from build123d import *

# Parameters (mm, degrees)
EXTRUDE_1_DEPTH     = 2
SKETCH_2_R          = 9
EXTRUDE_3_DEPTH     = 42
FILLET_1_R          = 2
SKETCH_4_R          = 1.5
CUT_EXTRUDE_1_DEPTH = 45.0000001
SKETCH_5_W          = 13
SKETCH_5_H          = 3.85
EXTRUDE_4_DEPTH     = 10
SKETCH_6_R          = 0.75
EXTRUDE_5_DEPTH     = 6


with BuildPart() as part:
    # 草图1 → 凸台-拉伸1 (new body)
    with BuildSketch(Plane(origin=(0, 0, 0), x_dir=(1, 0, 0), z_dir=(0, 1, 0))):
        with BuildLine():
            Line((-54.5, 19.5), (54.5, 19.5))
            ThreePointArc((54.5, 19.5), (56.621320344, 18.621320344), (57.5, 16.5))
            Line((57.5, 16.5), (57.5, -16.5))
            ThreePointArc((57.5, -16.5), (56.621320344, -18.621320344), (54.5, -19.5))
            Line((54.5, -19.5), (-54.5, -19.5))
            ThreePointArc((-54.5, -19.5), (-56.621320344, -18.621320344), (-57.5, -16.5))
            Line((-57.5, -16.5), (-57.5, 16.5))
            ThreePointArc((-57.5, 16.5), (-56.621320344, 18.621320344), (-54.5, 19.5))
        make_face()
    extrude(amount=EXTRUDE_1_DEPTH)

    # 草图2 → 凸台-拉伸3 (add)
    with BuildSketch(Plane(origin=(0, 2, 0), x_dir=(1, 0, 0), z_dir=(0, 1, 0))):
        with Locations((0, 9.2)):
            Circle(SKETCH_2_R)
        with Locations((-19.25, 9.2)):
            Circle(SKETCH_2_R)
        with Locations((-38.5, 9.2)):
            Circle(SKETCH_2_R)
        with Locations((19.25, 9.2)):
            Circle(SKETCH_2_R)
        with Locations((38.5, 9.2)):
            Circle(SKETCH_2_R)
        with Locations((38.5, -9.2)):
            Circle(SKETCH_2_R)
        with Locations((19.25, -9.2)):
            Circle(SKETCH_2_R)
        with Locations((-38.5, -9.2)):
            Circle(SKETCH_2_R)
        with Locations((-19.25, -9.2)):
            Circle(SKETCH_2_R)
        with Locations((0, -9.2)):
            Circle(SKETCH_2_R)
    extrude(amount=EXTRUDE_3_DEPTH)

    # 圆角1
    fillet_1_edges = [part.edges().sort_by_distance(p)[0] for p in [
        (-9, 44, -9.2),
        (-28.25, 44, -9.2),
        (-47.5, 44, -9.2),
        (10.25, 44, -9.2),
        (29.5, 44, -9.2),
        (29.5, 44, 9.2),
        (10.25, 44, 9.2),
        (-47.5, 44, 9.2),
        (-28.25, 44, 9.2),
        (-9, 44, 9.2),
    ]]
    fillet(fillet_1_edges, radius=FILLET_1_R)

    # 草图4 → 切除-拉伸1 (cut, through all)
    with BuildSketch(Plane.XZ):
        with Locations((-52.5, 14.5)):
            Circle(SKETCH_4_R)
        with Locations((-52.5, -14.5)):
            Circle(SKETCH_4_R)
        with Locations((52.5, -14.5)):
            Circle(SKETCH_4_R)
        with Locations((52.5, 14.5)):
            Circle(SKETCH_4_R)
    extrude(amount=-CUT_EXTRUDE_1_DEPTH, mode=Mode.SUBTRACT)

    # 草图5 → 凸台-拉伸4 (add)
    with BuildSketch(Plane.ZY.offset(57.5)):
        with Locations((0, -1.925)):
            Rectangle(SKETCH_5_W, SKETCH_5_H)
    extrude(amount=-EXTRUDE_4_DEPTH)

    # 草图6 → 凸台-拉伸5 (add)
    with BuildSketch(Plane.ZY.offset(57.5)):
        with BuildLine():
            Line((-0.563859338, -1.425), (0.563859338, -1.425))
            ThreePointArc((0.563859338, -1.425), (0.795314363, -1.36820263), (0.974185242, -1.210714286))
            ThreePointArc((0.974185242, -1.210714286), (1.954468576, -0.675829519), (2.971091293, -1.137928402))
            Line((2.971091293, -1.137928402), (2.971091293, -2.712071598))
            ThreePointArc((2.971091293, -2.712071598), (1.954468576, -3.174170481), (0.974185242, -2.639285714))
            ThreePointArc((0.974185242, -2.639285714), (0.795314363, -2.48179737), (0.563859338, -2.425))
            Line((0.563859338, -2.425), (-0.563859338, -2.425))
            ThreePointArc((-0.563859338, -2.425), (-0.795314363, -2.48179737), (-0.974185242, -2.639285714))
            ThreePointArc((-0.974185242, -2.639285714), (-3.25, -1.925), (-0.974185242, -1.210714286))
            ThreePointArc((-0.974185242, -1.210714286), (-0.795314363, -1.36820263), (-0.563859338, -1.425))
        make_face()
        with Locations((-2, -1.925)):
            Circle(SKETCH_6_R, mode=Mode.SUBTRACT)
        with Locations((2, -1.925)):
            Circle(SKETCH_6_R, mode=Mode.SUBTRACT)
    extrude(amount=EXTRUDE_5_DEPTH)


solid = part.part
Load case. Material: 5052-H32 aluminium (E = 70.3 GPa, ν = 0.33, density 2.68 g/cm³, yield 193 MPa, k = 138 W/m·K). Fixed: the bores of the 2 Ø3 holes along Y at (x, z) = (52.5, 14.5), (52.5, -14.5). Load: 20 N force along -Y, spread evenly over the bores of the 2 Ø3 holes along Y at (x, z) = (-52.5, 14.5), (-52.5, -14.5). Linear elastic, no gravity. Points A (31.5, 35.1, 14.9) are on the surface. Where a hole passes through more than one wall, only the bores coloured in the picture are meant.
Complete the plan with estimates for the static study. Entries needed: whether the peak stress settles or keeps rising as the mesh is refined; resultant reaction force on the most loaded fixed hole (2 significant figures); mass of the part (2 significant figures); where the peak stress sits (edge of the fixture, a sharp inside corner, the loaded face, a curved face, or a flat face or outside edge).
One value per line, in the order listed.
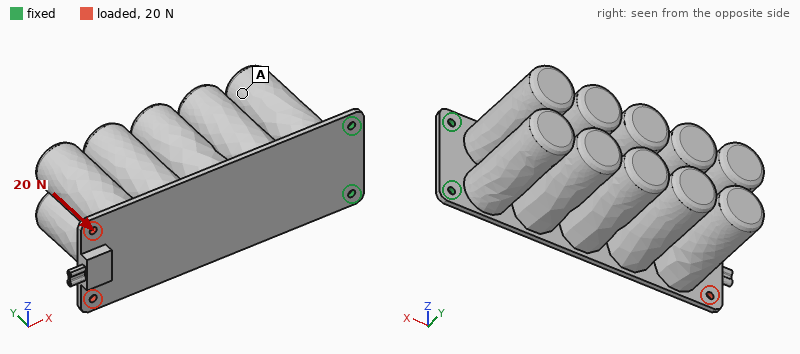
keeps rising
11 N
310 g
edge of the fixture
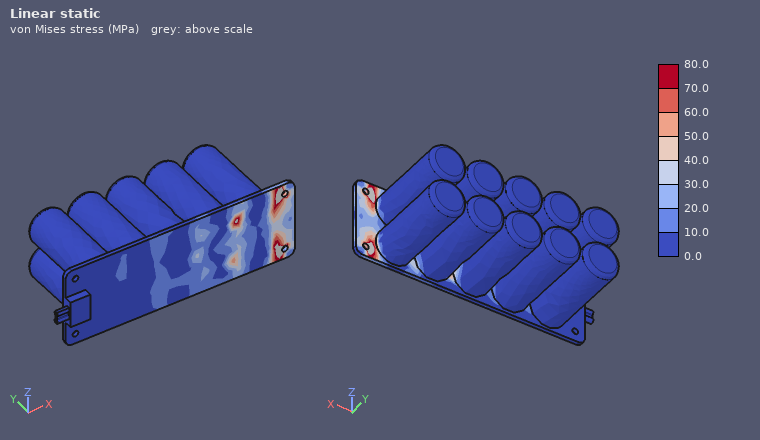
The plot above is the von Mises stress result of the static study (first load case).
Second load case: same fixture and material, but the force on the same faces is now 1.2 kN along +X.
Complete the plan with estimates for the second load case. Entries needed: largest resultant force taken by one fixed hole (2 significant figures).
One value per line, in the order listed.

610 N
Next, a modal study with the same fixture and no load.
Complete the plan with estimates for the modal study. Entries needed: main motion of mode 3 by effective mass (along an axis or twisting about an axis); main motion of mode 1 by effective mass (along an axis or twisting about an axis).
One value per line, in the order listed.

along Z
along Y
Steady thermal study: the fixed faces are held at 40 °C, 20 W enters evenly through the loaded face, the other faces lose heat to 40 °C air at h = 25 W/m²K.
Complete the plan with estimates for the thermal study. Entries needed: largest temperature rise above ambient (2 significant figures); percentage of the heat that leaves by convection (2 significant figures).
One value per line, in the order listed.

64 K
78 %
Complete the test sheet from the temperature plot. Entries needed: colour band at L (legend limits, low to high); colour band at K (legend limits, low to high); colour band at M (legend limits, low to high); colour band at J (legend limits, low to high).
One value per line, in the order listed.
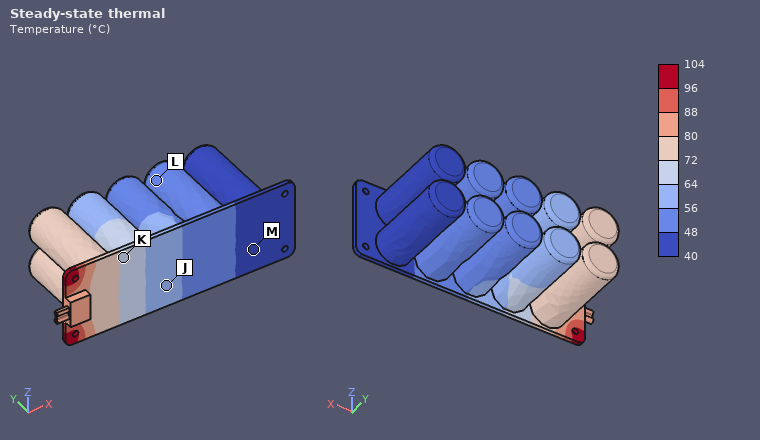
48 to 56 °C
64 to 72 °C
40 to 48 °C
56 to 64 °C
